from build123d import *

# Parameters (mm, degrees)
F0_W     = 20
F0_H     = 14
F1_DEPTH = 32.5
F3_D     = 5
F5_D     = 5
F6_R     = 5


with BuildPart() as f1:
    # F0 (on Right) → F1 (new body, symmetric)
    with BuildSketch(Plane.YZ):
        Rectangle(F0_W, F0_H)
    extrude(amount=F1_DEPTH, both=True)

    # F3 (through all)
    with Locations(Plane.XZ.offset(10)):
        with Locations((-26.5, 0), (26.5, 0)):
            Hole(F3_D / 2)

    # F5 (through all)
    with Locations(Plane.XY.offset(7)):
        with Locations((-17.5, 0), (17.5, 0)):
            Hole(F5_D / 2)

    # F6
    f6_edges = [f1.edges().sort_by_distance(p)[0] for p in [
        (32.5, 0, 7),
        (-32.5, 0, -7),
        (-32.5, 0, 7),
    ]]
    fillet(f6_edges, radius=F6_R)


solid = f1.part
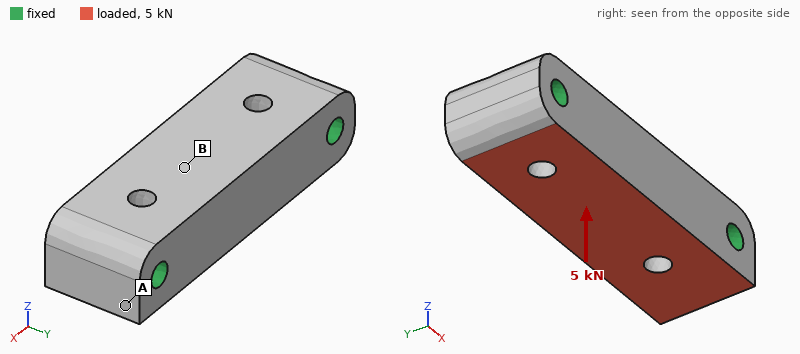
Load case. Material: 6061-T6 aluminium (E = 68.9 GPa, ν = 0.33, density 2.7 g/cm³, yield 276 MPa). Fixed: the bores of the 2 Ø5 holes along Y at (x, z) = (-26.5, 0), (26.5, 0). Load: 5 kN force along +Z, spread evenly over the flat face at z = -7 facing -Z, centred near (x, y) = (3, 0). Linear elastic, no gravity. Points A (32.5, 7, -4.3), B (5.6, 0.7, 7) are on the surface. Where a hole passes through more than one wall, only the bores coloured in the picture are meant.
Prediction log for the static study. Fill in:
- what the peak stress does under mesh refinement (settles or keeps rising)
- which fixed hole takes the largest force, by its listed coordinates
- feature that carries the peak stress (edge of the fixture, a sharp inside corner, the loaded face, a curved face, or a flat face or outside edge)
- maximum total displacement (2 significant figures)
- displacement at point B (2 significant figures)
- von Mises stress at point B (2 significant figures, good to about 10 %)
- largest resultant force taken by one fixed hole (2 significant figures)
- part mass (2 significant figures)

keeps rising
(26.5, 0)
edge of the fixture
14 µm
12 µm
18 MPa
2.7 kN
45 g
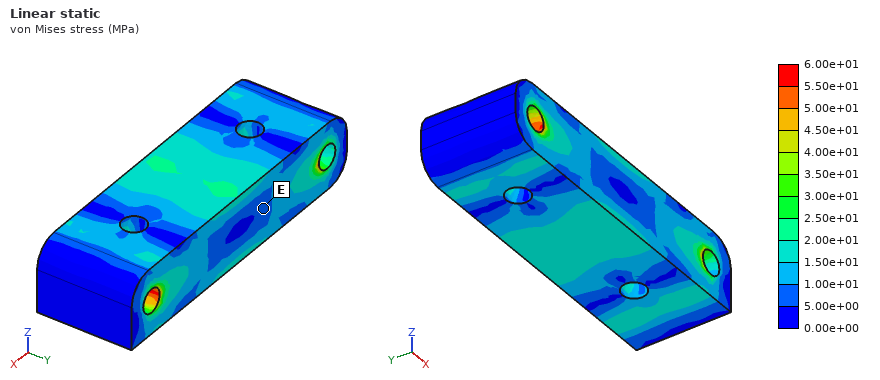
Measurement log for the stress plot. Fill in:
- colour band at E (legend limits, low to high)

5.00e+00 to 1.00e+01 MPa
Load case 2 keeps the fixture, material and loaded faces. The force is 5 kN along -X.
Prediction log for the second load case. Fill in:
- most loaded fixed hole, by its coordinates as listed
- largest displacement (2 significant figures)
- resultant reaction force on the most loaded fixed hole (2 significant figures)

(26.5, 0)
2.8 µm
2.7 kN
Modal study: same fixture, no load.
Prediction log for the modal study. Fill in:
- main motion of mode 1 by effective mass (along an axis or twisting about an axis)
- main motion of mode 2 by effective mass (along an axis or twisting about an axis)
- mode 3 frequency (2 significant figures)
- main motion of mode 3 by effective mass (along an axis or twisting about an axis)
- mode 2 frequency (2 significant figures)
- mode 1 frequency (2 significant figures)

along Z
along Y
25 kHz
twisting about X
21 kHz
16 kHz
